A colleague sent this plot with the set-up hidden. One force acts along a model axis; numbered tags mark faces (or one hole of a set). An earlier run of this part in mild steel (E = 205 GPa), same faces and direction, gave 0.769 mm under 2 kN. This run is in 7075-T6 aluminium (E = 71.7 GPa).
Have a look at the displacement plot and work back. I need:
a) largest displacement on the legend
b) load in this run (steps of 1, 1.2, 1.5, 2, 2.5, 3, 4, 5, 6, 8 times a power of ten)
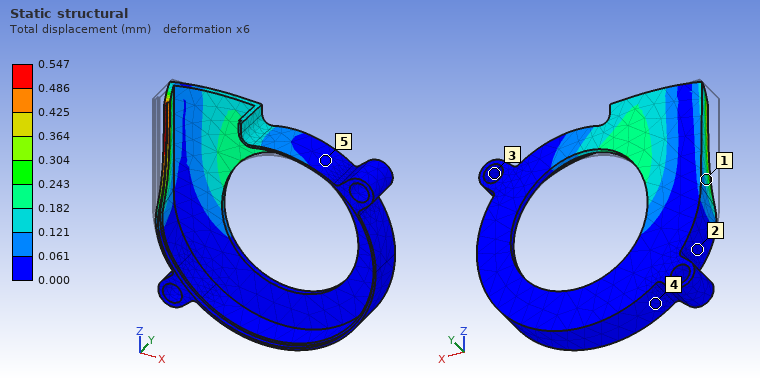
0.547 mm
500 N
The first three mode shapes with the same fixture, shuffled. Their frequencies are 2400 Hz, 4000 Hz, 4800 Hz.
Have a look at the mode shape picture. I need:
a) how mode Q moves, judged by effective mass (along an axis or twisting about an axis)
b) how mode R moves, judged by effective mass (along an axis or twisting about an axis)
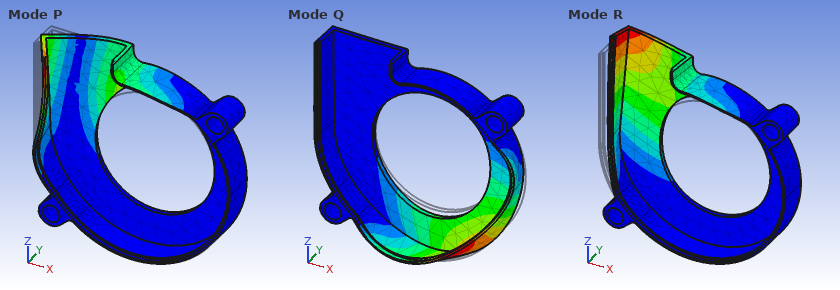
along Y
along Y
